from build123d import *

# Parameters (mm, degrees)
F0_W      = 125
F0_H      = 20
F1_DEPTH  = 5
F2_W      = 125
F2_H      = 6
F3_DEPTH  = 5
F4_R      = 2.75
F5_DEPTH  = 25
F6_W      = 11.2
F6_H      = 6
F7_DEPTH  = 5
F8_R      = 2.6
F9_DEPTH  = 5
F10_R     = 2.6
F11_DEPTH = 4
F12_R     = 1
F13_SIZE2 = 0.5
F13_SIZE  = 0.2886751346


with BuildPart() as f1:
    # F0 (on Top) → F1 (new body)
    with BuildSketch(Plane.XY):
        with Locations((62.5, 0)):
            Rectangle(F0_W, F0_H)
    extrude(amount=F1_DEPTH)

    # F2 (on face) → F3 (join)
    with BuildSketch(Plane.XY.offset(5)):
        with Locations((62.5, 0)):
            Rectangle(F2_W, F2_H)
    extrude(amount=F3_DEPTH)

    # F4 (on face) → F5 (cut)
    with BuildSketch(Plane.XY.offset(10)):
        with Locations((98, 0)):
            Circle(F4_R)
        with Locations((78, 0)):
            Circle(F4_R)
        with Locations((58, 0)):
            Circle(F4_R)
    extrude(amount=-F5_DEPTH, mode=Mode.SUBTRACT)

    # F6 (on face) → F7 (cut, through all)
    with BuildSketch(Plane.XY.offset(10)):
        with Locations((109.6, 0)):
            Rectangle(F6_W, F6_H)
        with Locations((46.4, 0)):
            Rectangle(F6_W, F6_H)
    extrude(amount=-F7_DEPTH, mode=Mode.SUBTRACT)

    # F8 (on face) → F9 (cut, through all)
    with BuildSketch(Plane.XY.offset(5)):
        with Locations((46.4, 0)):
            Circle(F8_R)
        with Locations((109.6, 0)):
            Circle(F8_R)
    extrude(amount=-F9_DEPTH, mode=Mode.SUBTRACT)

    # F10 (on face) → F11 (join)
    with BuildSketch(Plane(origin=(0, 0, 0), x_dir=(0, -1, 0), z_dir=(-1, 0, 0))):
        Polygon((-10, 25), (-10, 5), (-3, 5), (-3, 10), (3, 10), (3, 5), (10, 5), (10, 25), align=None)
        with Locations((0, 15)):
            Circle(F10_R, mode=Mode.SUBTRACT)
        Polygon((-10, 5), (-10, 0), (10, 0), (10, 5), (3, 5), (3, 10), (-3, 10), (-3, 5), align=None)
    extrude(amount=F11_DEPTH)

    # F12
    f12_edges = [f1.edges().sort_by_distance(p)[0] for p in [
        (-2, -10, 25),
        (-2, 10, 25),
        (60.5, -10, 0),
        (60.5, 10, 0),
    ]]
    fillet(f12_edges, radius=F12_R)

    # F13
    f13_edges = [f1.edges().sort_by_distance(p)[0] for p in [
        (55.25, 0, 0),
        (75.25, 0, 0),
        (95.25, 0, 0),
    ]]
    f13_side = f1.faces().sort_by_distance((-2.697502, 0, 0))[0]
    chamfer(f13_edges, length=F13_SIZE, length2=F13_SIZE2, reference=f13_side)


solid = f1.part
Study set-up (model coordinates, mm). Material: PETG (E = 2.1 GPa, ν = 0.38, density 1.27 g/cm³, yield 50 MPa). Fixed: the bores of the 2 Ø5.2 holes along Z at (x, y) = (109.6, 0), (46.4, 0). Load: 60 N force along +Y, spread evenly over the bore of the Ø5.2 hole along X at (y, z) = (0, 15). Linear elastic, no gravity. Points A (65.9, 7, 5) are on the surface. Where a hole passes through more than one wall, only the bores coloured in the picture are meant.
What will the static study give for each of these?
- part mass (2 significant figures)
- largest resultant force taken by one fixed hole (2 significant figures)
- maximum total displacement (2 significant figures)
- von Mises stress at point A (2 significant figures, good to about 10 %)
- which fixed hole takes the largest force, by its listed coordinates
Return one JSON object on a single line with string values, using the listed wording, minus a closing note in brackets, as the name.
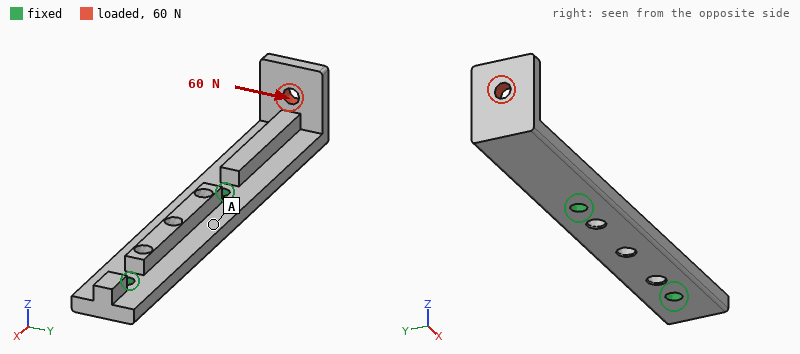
{"part mass": "21 g", "largest resultant force taken by one fixed hole": "85 N", "maximum total displacement": "1.5 mm", "von Mises stress at point A": "1.7 MPa", "which fixed hole takes the largest force, by its listed coordinates": "(46.4, 0)"}
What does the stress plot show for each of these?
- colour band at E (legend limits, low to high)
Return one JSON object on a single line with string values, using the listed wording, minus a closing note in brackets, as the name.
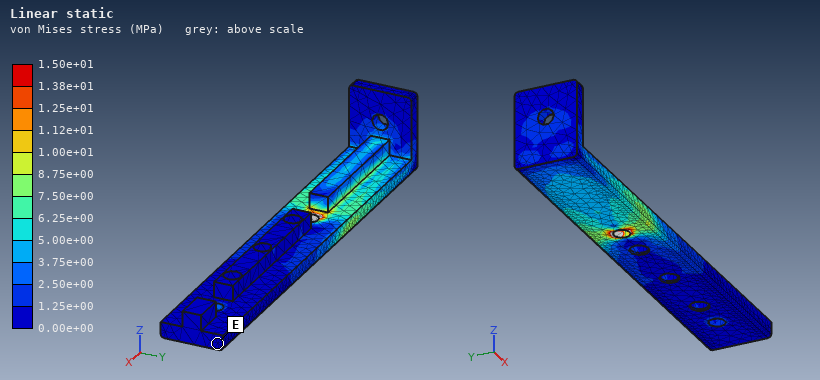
{"colour band at E": "0.00e+00 to 1.25e+00 MPa"}
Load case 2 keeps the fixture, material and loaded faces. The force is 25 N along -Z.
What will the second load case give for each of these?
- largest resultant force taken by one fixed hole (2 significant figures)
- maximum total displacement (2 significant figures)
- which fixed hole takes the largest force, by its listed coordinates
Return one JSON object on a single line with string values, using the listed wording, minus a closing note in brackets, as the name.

{"largest resultant force taken by one fixed hole": "26 N", "maximum total displacement": "1.4 mm", "which fixed hole takes the largest force, by its listed coordinates": "(46.4, 0)"}
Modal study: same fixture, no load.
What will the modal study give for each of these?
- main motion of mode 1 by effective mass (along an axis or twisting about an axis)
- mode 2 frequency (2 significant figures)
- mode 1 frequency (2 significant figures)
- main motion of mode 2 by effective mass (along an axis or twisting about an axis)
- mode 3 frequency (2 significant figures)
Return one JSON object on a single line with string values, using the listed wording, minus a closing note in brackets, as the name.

{"main motion of mode 1 by effective mass": "along Z", "mode 2 frequency": "690 Hz", "mode 1 frequency": "340 Hz", "main motion of mode 2 by effective mass": "along Y", "mode 3 frequency": "1200 Hz"}
